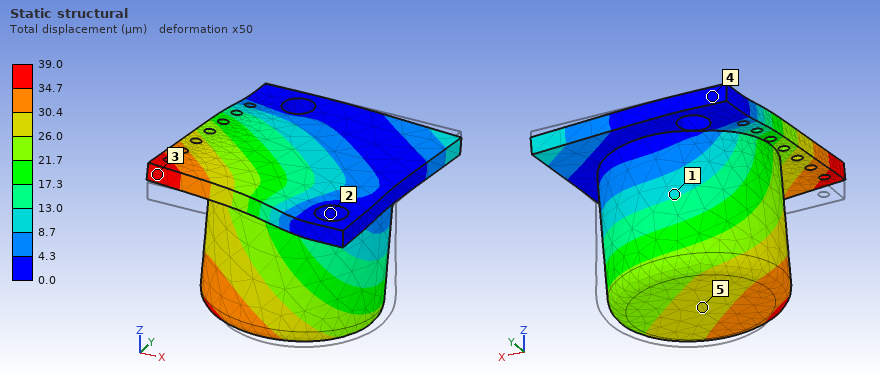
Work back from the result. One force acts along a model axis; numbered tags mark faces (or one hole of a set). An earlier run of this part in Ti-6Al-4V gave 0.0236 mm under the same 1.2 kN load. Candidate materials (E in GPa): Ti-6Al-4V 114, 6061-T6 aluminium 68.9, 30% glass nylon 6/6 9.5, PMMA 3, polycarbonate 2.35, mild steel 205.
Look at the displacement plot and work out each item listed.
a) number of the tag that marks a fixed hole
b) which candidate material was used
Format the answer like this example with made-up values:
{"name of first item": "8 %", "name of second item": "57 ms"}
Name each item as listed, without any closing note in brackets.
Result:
{"number of the tag that marks a fixed hole": "2", "which candidate material was used": "6061-T6 aluminium"}
